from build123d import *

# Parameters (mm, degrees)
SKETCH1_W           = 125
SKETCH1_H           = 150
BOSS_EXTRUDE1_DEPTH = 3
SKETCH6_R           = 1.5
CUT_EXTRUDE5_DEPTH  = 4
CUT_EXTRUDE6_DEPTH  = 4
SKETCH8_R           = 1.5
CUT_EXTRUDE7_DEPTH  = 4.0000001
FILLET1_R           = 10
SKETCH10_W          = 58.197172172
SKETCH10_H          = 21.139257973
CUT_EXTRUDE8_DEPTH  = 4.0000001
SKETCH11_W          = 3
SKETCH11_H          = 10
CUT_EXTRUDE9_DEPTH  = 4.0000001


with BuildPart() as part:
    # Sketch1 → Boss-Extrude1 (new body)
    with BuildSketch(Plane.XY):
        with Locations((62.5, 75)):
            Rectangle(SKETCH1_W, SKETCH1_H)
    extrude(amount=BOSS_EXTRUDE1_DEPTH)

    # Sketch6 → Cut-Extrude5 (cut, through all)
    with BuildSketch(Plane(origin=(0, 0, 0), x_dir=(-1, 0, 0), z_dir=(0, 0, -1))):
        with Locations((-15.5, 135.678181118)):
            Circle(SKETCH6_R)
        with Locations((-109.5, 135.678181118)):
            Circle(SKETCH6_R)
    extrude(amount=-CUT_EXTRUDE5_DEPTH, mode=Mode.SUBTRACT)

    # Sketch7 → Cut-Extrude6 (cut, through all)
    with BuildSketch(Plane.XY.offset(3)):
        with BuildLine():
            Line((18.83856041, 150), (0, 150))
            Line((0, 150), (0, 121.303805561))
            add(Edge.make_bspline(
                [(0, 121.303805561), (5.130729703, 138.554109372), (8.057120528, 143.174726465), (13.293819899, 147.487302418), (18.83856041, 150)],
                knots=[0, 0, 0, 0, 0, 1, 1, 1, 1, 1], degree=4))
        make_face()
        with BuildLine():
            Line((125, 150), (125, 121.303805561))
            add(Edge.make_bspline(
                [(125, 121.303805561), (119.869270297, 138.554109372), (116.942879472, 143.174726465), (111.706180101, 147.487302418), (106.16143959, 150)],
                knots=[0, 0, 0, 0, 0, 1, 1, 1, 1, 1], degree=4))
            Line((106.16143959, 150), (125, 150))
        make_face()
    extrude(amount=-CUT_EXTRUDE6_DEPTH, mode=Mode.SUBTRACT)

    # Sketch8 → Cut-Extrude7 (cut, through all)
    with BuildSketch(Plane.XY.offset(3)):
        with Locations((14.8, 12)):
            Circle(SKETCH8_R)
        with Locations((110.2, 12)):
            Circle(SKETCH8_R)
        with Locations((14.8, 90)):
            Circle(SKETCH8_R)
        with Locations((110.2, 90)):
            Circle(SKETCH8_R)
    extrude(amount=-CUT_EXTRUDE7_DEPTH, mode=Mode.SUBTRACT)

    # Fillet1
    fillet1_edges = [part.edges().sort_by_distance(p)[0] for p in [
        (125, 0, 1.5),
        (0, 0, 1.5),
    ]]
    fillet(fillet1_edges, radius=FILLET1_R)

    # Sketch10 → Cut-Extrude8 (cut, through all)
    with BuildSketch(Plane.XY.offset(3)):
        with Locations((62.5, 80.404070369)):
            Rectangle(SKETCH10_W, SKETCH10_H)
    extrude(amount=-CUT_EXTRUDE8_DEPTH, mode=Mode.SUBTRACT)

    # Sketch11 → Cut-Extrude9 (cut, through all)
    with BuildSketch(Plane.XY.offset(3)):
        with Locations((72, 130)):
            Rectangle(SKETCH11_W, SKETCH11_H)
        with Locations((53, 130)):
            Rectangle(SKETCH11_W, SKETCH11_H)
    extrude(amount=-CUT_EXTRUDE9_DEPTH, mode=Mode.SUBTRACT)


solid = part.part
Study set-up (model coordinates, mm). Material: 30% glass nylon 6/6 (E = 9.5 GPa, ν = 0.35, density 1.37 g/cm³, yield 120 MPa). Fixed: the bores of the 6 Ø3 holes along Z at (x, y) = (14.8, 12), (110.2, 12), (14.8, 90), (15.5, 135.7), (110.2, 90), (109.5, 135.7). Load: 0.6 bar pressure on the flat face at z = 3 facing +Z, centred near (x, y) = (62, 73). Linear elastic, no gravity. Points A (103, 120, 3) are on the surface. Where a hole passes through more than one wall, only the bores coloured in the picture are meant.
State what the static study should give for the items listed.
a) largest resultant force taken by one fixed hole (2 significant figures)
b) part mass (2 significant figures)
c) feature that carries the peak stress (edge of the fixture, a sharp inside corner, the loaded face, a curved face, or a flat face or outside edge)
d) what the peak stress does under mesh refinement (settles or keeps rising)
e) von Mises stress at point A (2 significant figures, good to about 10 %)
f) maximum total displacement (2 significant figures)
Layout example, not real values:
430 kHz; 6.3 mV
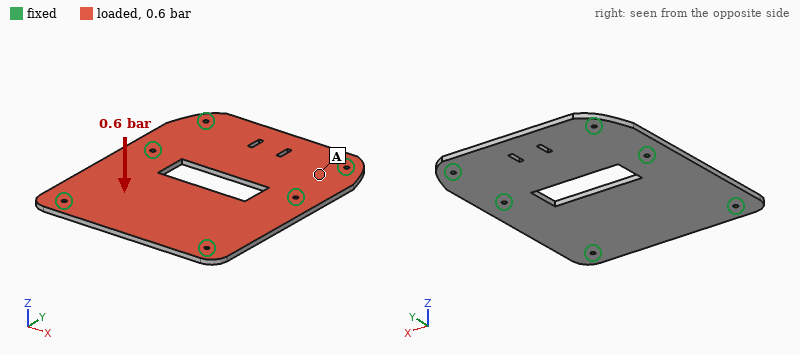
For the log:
210 N; 70 g; edge of the fixture; keeps rising; 10 MPa; 1.3 mm
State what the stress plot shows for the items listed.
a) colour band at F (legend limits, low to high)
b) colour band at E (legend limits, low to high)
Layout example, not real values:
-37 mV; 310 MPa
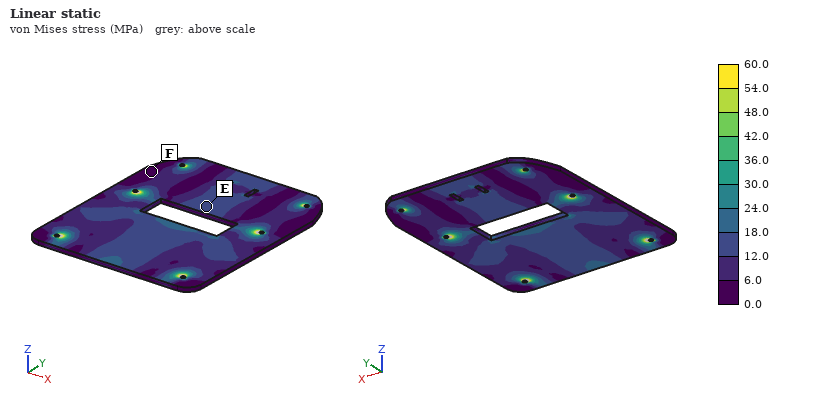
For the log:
0.0 to 6.0 MPa; 12.0 to 18.0 MPa
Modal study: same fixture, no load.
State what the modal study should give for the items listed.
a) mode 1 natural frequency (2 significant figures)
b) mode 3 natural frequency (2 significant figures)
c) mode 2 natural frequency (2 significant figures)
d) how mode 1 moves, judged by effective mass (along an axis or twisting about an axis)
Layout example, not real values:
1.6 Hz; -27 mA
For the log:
680 Hz; 1100 Hz; 840 Hz; along Z
